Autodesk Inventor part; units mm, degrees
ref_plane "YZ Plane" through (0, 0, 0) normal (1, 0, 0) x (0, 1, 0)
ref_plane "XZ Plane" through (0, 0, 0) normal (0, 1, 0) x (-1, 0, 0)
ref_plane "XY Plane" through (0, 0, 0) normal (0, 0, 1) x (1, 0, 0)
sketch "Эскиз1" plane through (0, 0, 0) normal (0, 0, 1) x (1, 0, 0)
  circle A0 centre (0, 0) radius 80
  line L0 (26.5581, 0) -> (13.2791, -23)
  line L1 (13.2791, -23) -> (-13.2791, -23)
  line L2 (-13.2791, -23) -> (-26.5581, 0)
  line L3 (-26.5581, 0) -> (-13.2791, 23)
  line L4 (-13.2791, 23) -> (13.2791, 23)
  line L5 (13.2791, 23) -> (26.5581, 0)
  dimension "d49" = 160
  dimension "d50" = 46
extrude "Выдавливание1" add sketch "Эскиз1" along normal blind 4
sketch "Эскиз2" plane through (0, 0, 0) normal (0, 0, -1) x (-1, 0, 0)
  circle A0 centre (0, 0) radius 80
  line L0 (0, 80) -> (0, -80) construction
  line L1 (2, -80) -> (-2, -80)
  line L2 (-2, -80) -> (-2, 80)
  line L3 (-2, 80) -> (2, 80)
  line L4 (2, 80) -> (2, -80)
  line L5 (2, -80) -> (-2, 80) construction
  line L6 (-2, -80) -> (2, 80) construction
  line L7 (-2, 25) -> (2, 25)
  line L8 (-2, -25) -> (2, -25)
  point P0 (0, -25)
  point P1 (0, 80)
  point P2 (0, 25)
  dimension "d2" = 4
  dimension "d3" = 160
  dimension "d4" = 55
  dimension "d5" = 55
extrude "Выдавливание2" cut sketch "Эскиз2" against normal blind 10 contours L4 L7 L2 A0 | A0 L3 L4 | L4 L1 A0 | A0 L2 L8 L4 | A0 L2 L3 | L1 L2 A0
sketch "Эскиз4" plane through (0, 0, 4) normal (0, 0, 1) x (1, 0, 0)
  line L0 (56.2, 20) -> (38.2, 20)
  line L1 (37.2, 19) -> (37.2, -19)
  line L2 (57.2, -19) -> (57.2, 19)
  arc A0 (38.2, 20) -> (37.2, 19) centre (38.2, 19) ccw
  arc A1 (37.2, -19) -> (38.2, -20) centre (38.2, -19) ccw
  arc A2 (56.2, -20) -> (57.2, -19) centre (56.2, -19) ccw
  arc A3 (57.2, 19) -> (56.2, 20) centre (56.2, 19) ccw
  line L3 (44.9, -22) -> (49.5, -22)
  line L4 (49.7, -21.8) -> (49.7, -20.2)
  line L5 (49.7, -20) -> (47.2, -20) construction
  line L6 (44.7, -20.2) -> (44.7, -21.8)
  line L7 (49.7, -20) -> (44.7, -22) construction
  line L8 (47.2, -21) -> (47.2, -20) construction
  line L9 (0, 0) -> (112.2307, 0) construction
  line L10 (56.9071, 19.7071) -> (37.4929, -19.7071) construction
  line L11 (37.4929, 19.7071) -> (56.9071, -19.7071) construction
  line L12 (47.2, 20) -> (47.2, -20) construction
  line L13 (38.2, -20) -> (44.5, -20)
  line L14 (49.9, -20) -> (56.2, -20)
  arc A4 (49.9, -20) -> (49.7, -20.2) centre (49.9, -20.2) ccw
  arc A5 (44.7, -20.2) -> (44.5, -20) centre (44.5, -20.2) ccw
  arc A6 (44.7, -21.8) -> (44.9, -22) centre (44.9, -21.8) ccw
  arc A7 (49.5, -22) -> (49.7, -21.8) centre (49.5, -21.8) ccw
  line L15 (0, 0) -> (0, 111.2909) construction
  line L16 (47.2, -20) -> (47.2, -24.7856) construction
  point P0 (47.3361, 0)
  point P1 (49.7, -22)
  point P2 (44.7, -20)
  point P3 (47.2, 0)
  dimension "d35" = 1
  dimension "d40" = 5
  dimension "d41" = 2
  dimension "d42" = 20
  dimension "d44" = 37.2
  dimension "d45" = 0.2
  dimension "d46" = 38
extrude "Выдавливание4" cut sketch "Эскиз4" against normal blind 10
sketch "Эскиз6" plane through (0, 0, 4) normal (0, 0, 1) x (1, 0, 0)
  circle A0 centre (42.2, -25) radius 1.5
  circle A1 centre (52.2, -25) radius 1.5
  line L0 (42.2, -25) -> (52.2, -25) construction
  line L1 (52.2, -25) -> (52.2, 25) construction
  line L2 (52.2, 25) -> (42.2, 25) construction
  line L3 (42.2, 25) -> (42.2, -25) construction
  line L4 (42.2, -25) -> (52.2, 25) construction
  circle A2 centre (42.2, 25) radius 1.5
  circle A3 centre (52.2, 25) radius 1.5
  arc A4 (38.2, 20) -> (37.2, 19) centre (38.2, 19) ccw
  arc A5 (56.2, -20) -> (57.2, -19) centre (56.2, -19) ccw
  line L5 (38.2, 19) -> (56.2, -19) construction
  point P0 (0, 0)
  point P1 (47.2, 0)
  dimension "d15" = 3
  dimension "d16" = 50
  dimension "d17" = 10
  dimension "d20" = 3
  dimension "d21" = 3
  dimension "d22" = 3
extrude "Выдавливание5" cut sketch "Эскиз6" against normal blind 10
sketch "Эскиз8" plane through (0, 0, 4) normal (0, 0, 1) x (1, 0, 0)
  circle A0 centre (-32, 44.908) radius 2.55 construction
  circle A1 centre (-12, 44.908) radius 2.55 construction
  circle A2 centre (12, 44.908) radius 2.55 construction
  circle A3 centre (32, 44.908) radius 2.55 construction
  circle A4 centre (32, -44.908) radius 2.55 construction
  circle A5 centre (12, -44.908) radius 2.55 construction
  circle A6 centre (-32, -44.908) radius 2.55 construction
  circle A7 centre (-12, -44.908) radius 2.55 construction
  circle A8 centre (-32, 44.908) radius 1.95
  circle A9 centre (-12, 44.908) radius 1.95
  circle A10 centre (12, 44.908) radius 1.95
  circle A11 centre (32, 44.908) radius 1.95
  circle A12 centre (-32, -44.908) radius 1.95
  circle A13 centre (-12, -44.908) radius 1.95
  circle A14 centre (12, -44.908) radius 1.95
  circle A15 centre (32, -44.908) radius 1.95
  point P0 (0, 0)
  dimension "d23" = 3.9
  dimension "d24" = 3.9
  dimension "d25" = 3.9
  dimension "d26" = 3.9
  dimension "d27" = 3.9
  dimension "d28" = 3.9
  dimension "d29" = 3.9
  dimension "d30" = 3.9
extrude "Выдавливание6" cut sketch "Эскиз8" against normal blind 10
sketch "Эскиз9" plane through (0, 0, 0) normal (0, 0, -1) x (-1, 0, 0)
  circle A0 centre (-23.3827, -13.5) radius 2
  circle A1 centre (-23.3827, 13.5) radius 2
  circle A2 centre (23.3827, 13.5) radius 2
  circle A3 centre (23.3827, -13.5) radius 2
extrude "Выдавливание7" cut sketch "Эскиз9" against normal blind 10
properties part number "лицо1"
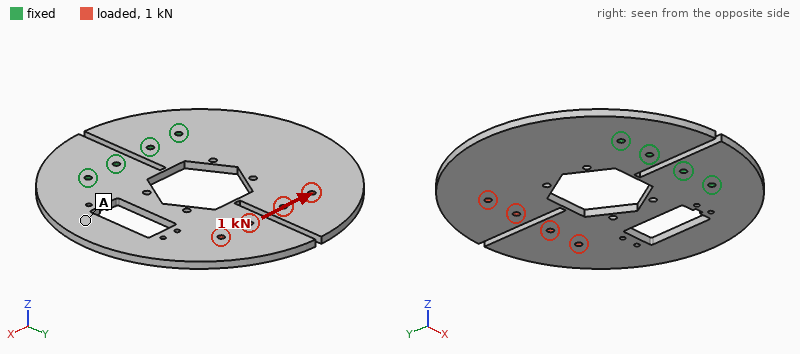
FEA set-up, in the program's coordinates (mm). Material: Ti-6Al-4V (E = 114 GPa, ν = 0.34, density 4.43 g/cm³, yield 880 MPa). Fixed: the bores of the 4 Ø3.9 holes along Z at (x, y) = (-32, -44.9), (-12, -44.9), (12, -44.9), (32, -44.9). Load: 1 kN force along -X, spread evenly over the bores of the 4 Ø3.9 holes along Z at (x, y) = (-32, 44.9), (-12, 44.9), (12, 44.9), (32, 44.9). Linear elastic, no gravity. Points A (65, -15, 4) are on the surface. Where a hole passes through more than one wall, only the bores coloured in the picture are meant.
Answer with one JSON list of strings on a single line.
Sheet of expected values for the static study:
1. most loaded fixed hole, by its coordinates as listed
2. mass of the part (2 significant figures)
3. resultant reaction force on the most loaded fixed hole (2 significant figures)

["(-32, -44.9)", "300 g", "2.0 kN"]
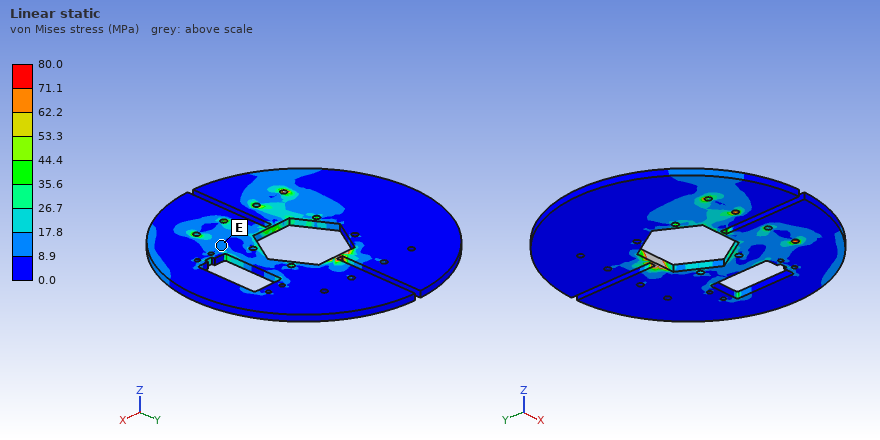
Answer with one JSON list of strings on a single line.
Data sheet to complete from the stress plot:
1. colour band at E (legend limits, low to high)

["8.9 to 17.8 MPa"]
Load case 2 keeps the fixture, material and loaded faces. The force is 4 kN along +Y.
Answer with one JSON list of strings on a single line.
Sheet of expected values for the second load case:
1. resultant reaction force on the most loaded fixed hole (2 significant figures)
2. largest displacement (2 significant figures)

["1.7 kN", "52 µm"]
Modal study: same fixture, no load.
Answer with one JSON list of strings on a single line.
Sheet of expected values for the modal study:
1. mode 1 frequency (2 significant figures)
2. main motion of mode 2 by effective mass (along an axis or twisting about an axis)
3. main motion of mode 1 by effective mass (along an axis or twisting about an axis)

["210 Hz", "twisting about Y", "along Z"]
